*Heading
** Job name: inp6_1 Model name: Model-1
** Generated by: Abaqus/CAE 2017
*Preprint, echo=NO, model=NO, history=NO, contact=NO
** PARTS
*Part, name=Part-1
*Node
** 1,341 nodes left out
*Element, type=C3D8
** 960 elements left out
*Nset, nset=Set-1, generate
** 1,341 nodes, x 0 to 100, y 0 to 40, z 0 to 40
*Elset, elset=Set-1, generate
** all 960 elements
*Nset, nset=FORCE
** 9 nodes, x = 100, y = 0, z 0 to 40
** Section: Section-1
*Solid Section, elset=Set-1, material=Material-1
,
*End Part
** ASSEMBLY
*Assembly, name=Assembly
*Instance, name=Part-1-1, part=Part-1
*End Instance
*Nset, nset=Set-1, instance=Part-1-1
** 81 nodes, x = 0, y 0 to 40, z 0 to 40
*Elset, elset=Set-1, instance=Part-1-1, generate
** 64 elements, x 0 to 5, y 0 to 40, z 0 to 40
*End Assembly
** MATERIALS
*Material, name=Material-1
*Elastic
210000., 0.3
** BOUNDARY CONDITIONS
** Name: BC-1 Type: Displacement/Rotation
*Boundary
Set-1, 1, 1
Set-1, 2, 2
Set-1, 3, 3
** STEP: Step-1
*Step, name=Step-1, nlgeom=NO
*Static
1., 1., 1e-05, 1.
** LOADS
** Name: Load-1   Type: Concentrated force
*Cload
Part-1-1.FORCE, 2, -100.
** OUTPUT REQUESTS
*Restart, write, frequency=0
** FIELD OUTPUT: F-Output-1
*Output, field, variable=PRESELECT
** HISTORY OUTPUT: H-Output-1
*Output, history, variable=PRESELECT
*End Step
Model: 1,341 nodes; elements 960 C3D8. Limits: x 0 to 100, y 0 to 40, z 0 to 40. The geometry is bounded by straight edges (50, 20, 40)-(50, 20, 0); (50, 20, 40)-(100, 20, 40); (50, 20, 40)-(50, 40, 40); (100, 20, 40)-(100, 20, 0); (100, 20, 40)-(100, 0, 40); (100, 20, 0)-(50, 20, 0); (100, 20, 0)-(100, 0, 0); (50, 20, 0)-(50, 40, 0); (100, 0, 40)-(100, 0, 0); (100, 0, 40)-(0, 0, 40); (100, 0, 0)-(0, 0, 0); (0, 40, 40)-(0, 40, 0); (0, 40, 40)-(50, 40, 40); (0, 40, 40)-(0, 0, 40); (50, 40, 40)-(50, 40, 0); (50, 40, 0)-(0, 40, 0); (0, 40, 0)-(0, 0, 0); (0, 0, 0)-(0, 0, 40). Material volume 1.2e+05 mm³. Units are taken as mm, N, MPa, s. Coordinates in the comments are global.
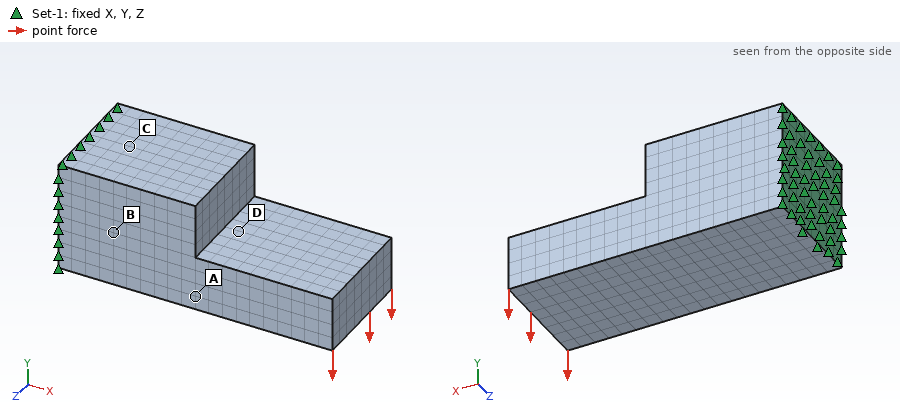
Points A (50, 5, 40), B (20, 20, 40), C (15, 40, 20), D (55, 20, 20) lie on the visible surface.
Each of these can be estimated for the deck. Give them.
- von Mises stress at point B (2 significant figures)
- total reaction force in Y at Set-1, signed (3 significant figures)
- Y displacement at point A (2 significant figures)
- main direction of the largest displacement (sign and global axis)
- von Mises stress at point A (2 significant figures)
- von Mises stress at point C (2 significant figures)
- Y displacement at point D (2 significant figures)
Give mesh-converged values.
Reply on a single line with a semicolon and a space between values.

1.9 MPa; 900 N; -0.0025 mm; -Y; 8.0 MPa; 6.7 MPa; -0.0036 mm
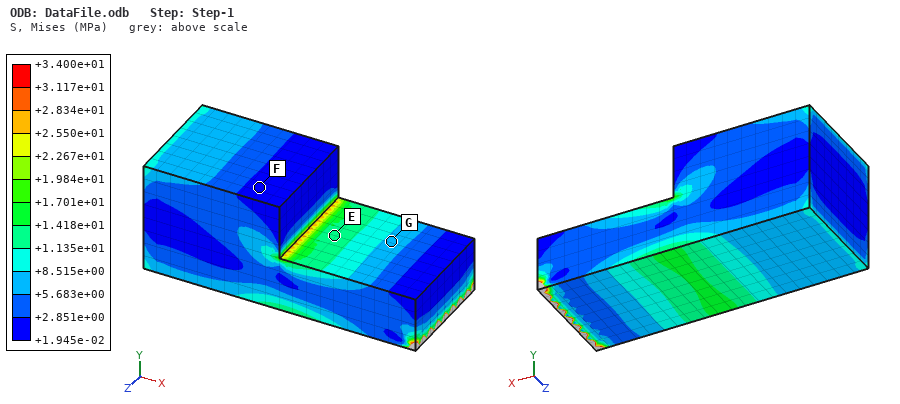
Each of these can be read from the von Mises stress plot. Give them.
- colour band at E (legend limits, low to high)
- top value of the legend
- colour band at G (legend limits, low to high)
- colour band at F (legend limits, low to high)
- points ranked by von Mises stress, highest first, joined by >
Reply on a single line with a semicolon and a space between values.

+1.135e+01 to +1.418e+01 MPa; +3.400e+01 MPa; +5.683e+00 to +8.515e+00 MPa; +1.945e-02 to +2.851e+00 MPa; E > G > F
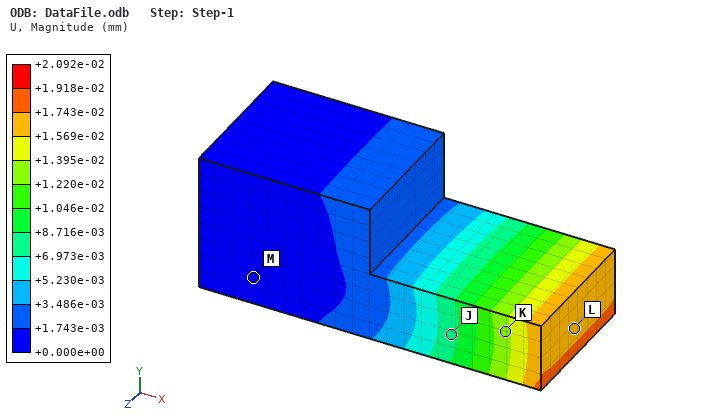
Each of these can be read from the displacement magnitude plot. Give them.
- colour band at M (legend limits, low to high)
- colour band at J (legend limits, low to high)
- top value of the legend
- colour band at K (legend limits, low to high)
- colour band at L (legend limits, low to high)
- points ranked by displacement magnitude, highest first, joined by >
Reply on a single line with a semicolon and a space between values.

+0.000e+00 to +1.743e-03 mm; +6.973e-03 to +8.716e-03 mm; +2.092e-02 mm; +1.220e-02 to +1.395e-02 mm; +1.569e-02 to +1.743e-02 mm; L > K > J > M
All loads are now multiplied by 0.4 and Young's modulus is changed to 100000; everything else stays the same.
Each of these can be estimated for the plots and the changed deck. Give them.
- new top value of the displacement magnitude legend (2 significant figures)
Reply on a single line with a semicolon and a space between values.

0.018 mm
